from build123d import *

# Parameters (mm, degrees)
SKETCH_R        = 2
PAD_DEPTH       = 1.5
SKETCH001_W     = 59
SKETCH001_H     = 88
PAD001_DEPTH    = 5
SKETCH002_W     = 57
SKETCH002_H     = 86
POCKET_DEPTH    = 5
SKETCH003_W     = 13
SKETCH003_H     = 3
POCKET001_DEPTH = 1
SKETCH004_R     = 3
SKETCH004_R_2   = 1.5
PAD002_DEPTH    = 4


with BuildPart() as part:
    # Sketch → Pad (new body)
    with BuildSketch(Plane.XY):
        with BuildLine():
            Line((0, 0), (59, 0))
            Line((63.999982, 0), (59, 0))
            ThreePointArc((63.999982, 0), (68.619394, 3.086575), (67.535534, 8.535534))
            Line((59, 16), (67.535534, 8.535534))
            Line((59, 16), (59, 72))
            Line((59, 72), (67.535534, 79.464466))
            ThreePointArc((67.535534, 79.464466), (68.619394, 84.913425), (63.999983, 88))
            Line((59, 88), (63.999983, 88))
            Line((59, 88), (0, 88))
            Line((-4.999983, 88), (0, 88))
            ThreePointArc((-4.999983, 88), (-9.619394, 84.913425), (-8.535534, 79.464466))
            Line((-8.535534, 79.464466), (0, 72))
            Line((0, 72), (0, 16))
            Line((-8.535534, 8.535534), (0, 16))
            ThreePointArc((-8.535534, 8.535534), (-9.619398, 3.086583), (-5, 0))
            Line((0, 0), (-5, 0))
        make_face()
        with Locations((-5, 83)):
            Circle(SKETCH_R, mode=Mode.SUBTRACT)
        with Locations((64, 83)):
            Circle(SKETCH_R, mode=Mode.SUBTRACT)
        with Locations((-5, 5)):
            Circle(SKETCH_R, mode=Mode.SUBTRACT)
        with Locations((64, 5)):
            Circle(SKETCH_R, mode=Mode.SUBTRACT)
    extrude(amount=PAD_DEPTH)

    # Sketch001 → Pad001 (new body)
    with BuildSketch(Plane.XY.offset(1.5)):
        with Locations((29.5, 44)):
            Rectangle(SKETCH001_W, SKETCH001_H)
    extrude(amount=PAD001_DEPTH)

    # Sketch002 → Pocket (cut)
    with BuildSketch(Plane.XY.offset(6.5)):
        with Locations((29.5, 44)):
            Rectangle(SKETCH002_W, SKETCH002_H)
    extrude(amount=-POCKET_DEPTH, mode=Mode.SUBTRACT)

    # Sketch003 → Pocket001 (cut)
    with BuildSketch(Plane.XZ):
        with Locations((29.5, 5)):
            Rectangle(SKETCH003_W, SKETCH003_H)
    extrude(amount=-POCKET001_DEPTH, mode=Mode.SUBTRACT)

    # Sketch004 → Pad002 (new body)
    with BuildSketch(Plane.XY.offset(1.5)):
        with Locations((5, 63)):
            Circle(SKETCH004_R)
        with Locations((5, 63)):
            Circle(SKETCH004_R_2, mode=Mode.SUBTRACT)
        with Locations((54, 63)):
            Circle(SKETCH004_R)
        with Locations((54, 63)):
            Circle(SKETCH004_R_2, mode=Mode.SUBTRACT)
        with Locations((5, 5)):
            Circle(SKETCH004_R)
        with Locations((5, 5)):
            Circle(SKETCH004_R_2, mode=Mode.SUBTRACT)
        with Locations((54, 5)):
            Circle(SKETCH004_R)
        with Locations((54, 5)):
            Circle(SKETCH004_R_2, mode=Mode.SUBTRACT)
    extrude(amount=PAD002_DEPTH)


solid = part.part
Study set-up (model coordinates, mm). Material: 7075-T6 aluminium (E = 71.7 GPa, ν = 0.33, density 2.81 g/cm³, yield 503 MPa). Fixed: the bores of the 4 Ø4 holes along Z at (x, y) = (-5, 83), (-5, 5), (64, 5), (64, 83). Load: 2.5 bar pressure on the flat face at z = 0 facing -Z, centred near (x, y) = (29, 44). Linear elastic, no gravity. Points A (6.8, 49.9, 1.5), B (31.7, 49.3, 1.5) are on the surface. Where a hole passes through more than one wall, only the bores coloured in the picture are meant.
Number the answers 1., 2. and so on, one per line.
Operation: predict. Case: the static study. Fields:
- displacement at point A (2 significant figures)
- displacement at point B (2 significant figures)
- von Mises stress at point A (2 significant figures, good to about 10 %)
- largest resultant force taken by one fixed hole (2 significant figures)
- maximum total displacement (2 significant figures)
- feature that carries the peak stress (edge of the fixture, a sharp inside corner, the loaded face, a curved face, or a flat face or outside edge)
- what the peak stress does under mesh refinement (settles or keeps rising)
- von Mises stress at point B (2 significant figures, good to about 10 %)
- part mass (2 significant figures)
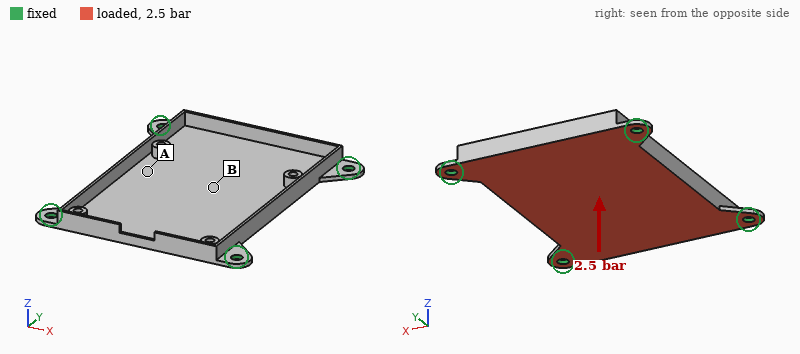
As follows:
1. 0.75 mm
2. 1.3 mm
3. 63 MPa
4. 460 N
5. 1.4 mm
6. edge of the fixture
7. keeps rising
8. 150 MPa
9. 28 g
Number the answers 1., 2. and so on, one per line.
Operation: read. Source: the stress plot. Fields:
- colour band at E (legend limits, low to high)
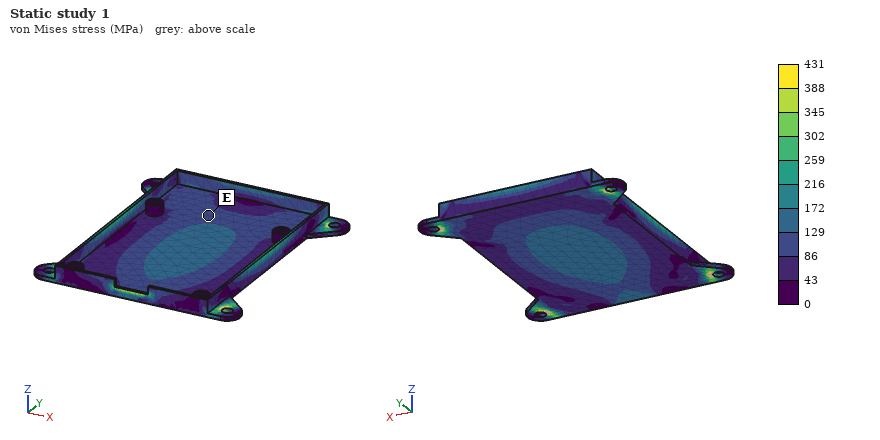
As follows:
1. 86 to 129 MPa
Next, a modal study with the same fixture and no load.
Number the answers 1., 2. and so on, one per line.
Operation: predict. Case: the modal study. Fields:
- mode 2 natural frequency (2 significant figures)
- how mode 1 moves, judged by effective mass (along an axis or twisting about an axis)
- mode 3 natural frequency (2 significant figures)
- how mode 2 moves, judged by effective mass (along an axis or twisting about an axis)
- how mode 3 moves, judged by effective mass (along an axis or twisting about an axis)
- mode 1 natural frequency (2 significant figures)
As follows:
1. 2300 Hz
2. along Z
3. 2700 Hz
4. twisting about X
5. twisting about Y
6. 1300 Hz
